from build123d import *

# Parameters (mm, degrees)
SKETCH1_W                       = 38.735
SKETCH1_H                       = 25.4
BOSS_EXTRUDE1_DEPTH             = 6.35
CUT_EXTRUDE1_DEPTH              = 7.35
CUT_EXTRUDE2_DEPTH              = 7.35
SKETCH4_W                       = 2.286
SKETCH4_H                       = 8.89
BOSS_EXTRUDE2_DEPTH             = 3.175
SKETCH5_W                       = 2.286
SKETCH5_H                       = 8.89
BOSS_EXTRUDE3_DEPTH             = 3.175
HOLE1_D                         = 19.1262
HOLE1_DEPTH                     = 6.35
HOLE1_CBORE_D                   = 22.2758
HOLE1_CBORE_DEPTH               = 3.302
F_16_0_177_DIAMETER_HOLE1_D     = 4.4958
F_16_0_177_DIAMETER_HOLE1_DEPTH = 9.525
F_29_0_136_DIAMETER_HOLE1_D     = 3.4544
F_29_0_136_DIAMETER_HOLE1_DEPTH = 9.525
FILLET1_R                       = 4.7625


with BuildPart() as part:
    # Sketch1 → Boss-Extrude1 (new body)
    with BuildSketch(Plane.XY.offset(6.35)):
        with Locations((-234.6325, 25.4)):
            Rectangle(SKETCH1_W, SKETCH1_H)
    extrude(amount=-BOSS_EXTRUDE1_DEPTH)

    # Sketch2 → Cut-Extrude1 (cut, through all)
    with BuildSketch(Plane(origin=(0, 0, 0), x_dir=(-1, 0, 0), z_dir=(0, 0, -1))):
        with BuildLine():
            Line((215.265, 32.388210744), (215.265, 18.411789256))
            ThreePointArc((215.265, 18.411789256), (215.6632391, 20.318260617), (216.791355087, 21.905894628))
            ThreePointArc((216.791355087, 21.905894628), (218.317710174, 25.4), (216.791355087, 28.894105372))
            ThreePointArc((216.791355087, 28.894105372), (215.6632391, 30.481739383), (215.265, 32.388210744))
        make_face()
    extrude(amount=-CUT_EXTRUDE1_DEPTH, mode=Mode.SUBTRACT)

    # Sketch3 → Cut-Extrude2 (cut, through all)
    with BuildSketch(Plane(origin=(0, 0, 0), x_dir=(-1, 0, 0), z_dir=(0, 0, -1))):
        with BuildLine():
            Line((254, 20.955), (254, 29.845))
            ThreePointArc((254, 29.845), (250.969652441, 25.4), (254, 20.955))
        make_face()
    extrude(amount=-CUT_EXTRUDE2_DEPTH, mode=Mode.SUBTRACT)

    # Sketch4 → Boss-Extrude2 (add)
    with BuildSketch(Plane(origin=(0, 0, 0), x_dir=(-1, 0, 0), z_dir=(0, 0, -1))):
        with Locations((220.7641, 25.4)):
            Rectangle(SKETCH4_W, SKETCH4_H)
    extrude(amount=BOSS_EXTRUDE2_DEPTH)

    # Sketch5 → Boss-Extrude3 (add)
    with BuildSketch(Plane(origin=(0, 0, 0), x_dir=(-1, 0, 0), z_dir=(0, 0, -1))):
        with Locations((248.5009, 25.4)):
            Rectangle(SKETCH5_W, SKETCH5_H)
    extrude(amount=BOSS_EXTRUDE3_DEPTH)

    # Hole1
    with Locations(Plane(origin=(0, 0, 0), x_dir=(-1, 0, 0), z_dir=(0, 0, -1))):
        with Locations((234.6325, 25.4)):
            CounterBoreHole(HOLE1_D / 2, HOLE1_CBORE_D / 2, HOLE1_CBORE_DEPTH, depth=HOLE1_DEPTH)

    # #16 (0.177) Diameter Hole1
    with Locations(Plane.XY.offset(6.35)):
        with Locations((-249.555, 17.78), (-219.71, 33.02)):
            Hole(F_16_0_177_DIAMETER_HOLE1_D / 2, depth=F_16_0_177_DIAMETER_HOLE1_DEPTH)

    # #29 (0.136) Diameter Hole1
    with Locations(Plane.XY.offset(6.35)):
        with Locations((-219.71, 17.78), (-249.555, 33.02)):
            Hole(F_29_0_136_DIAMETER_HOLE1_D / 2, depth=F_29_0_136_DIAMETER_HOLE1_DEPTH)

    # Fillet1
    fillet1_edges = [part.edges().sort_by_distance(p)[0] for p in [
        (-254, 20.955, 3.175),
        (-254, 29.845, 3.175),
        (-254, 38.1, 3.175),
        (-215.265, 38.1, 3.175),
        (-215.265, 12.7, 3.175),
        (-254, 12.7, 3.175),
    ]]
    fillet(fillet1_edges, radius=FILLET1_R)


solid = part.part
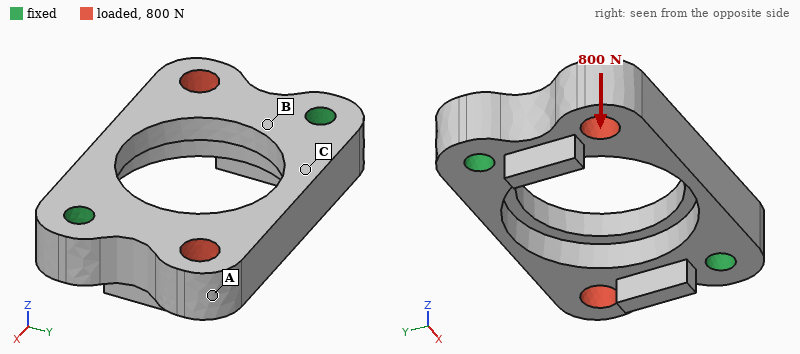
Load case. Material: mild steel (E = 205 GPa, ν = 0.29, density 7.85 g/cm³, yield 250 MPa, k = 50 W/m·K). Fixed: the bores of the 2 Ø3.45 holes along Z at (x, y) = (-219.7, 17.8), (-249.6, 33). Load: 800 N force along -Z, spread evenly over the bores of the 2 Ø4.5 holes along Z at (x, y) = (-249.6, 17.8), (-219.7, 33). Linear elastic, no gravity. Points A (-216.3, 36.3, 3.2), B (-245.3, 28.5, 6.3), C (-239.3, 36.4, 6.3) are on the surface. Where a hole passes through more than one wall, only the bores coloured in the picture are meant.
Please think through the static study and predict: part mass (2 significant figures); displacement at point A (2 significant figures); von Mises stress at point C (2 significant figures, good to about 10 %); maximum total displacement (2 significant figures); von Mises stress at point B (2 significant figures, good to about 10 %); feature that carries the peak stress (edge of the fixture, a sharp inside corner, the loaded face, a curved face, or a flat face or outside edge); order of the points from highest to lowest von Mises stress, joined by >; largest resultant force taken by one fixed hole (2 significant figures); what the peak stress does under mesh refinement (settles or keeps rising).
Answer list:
27 g
15 µm
27 MPa
16 µm
51 MPa
edge of the fixture
B > C > A
410 N
keeps rising
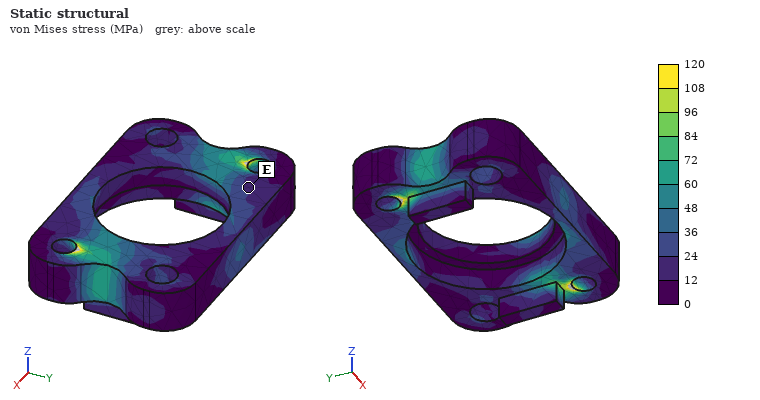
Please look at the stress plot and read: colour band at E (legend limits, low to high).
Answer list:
12 to 24 MPa
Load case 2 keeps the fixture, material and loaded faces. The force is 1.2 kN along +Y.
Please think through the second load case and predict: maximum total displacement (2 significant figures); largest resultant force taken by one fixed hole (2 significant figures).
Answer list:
1.8 µm
600 N
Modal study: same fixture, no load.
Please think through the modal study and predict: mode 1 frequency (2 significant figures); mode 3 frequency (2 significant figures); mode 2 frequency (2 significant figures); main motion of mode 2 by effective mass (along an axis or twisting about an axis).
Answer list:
13 kHz
27 kHz
14 kHz
along Z
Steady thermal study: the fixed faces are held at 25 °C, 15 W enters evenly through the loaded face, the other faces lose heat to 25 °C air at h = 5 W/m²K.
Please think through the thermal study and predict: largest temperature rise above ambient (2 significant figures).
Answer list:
41 K
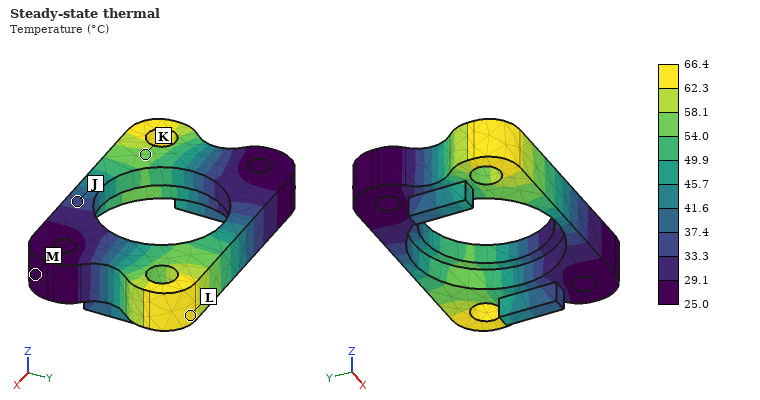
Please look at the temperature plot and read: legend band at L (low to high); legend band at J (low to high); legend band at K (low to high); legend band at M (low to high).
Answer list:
62.3 to 66.4 °C
33.3 to 37.4 °C
54.0 to 58.1 °C
25.0 to 29.1 °C
